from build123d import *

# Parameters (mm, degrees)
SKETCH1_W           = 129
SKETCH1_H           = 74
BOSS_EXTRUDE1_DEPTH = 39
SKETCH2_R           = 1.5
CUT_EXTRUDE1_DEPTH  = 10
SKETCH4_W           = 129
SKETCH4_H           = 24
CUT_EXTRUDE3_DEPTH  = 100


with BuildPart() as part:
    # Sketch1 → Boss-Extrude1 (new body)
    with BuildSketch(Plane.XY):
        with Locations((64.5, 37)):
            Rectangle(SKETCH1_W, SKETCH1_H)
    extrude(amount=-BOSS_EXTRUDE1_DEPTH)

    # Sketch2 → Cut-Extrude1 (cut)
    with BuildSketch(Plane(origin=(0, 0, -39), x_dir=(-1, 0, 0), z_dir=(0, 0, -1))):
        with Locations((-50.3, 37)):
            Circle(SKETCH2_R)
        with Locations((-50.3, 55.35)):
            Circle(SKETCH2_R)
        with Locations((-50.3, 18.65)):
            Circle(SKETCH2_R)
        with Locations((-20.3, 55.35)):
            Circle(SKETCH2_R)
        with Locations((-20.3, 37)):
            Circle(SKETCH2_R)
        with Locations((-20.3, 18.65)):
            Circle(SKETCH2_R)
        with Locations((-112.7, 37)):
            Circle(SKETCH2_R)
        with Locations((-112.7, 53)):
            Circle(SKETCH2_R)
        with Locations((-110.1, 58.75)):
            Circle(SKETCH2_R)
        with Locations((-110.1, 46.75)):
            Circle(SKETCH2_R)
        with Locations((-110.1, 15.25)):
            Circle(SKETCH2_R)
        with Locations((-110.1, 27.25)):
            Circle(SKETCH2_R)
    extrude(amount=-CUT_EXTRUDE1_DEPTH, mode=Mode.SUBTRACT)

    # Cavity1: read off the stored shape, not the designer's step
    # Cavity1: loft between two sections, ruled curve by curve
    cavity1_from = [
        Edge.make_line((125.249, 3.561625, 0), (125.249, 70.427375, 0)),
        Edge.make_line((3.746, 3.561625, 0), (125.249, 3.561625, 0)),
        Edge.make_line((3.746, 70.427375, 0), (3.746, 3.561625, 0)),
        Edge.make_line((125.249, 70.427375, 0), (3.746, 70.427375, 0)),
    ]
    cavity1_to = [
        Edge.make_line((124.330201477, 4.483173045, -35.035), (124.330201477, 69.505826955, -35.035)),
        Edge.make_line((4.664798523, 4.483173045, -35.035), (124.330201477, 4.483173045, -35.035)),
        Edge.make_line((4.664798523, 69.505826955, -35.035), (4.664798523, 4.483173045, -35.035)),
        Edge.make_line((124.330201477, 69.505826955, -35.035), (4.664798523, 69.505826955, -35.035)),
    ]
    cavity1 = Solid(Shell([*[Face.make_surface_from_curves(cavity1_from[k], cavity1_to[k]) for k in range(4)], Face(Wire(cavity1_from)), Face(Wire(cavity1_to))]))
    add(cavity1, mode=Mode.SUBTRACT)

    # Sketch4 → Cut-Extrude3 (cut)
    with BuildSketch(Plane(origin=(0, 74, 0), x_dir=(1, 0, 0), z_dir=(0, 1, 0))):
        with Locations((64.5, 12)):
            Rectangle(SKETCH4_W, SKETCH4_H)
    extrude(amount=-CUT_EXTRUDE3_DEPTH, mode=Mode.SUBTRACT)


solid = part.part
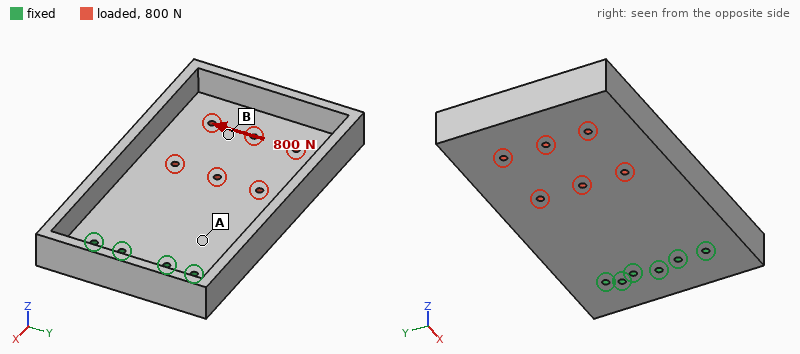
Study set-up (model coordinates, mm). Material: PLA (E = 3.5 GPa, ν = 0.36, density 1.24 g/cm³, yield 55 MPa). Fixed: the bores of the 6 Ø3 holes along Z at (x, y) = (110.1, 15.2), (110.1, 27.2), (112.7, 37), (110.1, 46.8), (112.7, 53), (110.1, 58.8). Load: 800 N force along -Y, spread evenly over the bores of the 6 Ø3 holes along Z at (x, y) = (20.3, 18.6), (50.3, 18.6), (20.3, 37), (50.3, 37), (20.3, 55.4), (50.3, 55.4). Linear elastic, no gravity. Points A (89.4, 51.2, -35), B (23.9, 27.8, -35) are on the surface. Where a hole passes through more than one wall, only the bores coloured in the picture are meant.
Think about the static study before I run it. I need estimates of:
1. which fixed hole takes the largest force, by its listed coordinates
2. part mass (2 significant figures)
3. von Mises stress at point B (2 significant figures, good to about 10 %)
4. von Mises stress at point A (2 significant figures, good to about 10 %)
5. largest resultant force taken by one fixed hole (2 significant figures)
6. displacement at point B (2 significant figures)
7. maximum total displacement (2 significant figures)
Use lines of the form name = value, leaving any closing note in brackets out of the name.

which fixed hole takes the largest force, by its listed coordinates = (110.1, 15.2)
part mass = 70 g
von Mises stress at point B = 4.0 MPa
von Mises stress at point A = 8.8 MPa
largest resultant force taken by one fixed hole = 1.2 kN
displacement at point B = 0.63 mm
maximum total displacement = 0.94 mm
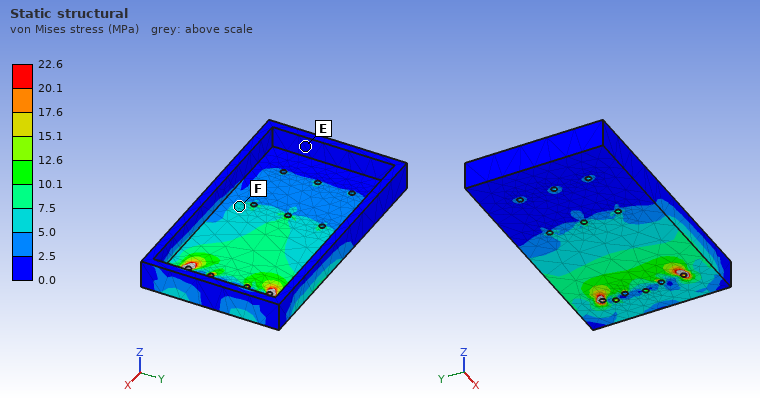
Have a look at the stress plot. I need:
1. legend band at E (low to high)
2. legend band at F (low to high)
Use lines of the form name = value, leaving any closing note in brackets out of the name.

legend band at E = 0.0 to 2.5 MPa
legend band at F = 5.0 to 7.5 MPa
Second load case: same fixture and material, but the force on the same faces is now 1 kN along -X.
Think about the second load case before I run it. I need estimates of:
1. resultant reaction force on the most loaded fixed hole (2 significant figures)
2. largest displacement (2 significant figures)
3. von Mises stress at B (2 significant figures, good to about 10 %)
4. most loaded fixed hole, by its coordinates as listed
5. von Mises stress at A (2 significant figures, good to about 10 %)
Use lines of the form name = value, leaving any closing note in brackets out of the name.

resultant reaction force on the most loaded fixed hole = 290 N
largest displacement = 0.31 mm
von Mises stress at B = 0.86 MPa
most loaded fixed hole, by its coordinates as listed = (110.1, 15.2)
von Mises stress at A = 3.5 MPa
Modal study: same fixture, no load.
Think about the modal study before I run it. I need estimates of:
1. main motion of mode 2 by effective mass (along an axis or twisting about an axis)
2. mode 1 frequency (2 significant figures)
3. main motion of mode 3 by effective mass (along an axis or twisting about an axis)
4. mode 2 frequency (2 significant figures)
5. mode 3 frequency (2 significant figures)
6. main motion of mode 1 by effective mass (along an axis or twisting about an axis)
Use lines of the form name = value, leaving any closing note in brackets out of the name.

main motion of mode 2 by effective mass = twisting about X
mode 1 frequency = 140 Hz
main motion of mode 3 by effective mass = along Y
mode 2 frequency = 280 Hz
mode 3 frequency = 860 Hz
main motion of mode 1 by effective mass = along Z
